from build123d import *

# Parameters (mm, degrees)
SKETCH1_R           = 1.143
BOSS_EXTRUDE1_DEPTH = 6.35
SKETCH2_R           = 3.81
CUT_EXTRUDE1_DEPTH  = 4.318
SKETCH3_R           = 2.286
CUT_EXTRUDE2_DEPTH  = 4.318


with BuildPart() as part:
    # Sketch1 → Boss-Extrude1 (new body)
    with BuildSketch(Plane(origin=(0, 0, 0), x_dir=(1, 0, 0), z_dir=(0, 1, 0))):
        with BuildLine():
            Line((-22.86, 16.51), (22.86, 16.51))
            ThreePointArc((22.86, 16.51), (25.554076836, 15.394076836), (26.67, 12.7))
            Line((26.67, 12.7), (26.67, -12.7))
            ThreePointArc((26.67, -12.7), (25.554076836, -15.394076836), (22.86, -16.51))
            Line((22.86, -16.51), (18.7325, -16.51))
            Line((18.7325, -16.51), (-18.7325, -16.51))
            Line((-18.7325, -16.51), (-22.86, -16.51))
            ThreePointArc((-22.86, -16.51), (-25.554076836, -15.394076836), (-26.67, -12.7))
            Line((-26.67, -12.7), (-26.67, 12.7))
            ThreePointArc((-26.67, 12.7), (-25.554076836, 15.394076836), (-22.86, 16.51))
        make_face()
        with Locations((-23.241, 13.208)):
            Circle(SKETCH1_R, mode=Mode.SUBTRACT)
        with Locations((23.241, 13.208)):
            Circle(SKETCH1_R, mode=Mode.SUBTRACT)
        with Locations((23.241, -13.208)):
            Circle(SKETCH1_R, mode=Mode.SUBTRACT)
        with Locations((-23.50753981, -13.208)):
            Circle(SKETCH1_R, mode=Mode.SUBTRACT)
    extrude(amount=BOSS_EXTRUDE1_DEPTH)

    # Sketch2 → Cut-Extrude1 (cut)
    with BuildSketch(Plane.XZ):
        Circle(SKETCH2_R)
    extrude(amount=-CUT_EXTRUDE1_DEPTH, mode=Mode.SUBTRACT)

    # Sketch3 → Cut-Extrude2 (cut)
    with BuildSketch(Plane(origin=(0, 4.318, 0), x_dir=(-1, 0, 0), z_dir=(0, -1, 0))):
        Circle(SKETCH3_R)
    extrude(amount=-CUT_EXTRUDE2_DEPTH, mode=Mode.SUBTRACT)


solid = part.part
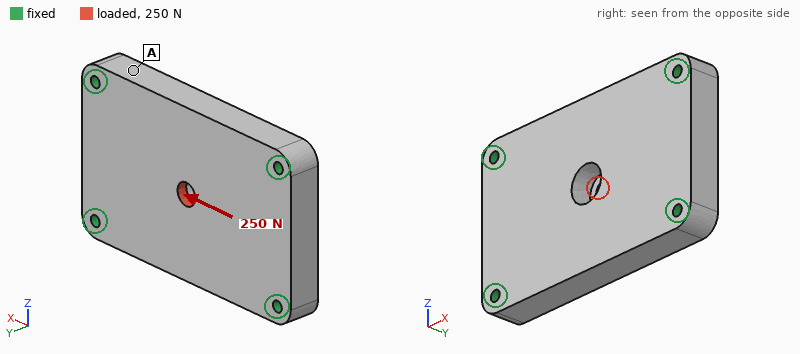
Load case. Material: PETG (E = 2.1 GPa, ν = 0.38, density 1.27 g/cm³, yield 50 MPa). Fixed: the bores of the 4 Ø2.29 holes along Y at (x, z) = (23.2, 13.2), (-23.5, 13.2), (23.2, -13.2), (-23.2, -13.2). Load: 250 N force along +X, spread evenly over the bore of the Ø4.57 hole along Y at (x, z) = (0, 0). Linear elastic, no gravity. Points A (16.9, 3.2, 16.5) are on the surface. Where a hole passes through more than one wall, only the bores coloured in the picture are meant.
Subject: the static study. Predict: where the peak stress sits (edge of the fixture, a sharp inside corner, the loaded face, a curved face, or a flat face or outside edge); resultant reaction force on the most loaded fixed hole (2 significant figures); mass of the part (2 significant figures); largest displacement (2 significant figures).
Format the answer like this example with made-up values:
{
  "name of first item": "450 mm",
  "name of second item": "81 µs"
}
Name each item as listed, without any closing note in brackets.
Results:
{
  "where the peak stress sits": "a sharp inside corner",
  "resultant reaction force on the most loaded fixed hole": "67 N",
  "mass of the part": "14 g",
  "largest displacement": "31 µm"
}
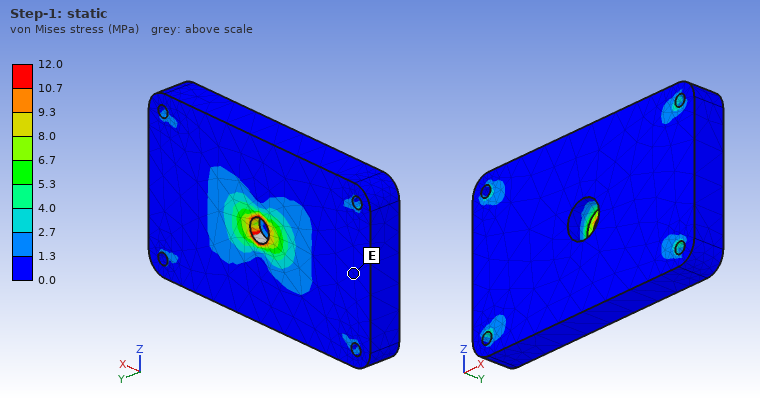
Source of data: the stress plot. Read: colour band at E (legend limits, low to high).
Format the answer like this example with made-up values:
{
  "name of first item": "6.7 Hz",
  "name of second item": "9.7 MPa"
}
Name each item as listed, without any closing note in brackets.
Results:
{
  "colour band at E": "0.0 to 1.3 MPa"
}
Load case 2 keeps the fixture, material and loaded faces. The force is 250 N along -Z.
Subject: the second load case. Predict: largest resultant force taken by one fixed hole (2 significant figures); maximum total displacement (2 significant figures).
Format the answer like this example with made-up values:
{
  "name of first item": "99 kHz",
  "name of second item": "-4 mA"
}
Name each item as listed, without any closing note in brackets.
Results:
{
  "largest resultant force taken by one fixed hole": "84 N",
  "maximum total displacement": "45 µm"
}
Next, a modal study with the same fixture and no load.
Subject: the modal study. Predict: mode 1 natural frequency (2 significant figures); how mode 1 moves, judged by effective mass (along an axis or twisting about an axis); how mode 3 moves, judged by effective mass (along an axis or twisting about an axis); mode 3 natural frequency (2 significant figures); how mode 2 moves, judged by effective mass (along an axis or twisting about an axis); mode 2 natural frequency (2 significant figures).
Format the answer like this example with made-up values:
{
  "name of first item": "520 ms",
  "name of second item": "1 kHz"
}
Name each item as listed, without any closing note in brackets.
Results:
{
  "mode 1 natural frequency": "2800 Hz",
  "how mode 1 moves, judged by effective mass": "along Y",
  "how mode 3 moves, judged by effective mass": "twisting about Z",
  "mode 3 natural frequency": "6800 Hz",
  "how mode 2 moves, judged by effective mass": "twisting about X",
  "mode 2 natural frequency": "4300 Hz"
}
